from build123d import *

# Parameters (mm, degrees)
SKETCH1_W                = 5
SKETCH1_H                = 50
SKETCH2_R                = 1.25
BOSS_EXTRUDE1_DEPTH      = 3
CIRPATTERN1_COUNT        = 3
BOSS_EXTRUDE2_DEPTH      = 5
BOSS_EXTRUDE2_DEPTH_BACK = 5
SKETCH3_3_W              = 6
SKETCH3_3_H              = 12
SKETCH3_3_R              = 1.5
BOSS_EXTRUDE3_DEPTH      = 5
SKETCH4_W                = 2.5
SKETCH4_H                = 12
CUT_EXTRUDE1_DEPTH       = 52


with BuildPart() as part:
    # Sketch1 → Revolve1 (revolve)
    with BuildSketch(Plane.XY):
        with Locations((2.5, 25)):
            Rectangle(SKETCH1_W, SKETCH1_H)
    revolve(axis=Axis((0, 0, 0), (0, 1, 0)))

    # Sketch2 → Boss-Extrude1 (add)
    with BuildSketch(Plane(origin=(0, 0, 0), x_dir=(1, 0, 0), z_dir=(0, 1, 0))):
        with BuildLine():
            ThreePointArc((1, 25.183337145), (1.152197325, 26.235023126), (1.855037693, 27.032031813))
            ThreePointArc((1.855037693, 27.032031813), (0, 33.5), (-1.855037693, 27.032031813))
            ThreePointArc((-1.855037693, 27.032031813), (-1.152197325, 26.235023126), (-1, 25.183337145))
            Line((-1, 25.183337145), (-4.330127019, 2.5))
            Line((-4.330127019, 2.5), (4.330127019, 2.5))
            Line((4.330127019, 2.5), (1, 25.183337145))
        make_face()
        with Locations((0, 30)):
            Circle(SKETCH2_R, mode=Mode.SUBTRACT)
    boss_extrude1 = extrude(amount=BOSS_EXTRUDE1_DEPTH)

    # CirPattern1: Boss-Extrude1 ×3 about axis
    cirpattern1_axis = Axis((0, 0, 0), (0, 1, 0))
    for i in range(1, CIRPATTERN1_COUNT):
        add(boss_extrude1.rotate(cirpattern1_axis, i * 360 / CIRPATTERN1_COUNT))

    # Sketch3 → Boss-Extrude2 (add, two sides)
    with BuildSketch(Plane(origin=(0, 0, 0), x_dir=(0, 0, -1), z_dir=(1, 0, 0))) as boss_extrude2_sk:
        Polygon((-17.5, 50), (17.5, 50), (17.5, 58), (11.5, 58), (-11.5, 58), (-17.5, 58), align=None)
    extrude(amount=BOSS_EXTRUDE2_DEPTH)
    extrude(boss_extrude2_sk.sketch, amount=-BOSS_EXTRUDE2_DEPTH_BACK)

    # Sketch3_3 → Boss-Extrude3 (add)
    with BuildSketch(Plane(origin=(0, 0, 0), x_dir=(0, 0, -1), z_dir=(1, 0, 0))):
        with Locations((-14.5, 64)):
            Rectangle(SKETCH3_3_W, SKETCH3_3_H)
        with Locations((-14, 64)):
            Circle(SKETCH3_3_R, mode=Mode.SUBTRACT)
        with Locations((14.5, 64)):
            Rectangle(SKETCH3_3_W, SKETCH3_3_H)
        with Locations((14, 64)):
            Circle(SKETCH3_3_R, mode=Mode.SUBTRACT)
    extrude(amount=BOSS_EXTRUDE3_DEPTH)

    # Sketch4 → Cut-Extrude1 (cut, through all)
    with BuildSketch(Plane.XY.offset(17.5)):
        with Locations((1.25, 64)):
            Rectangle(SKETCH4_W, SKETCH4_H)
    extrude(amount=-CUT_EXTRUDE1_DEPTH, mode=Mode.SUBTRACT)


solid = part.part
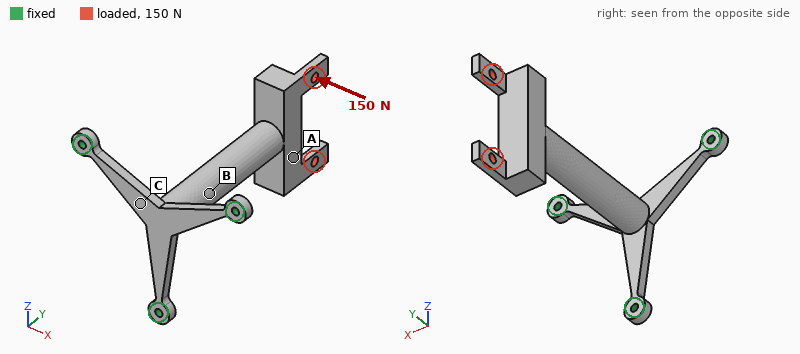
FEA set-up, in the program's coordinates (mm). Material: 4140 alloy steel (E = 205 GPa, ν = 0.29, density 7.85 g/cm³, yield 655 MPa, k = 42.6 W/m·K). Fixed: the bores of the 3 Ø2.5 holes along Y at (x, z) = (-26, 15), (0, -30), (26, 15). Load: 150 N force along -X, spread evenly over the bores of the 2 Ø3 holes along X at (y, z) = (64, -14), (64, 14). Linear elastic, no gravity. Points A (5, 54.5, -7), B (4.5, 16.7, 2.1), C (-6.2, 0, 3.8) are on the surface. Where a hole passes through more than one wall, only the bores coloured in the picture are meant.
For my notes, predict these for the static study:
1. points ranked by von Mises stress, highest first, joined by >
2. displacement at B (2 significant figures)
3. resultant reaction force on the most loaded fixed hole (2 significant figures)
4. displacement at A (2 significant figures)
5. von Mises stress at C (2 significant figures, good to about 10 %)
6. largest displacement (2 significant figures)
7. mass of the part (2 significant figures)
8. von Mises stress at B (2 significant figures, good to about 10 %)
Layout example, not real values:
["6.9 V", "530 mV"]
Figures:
["C > B > A", "0.16 mm", "240 N", "0.60 mm", "290 MPa", "0.81 mm", "65 g", "66 MPa"]
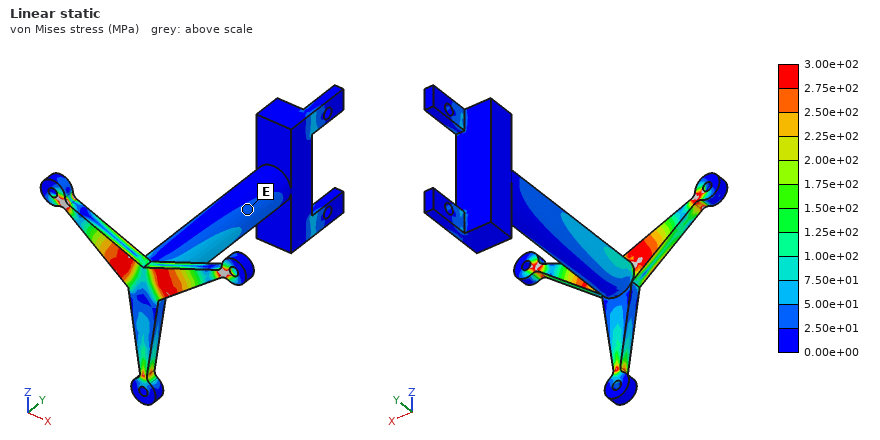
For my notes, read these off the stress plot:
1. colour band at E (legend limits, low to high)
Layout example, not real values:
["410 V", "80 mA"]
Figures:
["2.50e+01 to 5.00e+01 MPa"]
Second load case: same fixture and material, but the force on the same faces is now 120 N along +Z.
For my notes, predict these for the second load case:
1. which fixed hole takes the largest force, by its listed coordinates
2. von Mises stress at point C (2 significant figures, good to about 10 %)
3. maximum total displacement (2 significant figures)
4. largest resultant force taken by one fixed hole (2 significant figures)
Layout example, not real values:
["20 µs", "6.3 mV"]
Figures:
["(0, -30)", "140 MPa", "0.66 mm", "230 N"]
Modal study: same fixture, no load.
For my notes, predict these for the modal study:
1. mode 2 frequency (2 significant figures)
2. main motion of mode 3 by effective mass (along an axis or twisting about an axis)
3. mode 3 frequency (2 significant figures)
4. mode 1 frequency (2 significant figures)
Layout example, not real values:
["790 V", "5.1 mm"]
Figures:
["480 Hz", "along Y", "1400 Hz", "470 Hz"]
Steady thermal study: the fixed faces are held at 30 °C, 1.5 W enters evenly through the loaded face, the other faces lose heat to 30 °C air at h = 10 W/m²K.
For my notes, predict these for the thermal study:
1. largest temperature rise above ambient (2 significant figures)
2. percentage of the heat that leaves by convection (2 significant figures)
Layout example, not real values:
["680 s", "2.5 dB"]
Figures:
["37 K", "55 %"]
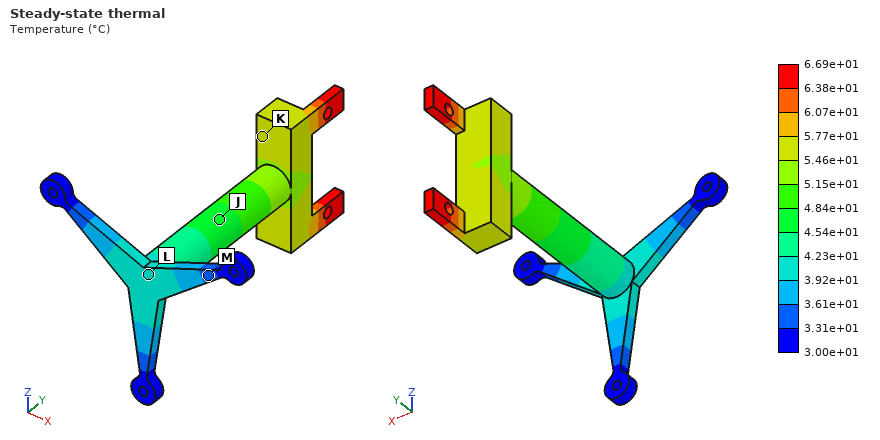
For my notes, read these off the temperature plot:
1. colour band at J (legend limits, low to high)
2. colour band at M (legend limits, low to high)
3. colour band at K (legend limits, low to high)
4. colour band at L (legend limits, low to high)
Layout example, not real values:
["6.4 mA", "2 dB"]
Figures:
["4.54e+01 to 4.84e+01 °C", "3.31e+01 to 3.61e+01 °C", "5.46e+01 to 5.77e+01 °C", "3.92e+01 to 4.23e+01 °C"]
